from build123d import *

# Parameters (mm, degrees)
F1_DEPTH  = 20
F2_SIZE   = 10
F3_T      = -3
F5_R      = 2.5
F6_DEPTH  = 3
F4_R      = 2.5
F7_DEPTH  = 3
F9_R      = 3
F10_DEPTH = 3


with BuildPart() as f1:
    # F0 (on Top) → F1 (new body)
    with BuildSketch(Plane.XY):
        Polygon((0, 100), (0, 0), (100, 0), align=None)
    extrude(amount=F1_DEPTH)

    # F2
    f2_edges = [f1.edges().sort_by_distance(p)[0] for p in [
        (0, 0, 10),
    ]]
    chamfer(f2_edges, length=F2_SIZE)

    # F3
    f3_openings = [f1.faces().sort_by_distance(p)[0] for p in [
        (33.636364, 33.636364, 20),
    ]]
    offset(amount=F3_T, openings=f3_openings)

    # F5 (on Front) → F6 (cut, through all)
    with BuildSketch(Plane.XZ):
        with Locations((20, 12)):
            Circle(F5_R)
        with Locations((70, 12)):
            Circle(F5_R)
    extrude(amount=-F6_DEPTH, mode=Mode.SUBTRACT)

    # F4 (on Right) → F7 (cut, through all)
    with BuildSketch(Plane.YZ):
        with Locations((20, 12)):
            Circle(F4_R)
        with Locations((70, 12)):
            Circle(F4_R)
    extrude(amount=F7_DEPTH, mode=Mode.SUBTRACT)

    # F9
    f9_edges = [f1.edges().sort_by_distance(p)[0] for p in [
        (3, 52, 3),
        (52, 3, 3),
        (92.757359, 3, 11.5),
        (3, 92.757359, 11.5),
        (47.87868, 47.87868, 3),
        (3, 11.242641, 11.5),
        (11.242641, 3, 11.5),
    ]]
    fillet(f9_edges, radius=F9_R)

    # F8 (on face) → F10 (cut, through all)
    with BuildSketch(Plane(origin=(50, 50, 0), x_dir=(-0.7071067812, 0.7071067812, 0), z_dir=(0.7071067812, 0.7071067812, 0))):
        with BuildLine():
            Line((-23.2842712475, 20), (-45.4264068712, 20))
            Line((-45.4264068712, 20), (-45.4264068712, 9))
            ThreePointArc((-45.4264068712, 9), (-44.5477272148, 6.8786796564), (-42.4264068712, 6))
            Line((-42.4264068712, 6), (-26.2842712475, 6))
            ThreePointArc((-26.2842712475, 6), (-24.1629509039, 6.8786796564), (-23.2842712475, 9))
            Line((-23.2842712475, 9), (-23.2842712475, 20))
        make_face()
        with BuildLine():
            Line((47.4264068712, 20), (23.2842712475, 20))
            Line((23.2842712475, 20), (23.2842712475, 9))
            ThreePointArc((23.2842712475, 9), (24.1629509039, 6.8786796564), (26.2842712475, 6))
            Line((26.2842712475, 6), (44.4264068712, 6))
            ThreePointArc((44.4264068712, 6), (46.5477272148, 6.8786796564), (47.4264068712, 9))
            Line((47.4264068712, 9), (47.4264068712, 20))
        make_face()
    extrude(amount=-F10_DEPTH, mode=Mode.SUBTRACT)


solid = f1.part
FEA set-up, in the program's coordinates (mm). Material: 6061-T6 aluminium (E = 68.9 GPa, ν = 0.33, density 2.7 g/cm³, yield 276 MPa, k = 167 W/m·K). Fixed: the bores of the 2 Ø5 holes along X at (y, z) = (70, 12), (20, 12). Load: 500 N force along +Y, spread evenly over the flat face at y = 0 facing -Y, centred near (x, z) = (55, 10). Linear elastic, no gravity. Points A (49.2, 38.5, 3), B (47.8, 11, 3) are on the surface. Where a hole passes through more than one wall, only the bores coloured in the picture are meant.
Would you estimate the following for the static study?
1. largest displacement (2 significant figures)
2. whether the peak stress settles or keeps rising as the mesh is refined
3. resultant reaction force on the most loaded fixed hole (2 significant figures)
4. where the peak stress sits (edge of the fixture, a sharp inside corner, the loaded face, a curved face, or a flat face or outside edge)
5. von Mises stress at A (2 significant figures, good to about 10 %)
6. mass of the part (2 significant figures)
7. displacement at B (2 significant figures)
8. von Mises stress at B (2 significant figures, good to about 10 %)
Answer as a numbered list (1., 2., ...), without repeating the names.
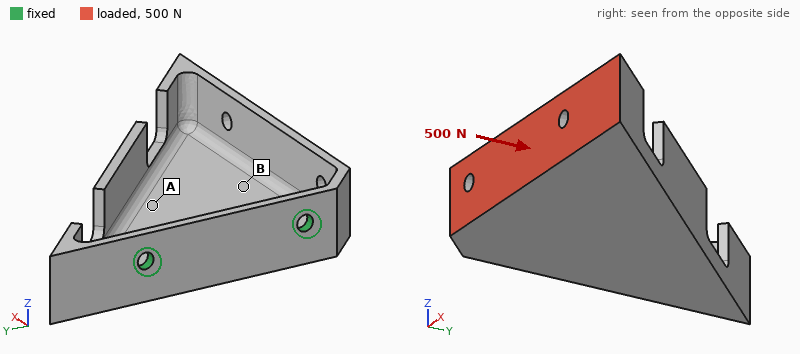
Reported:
1. 0.33 mm
2. keeps rising
3. 580 N
4. edge of the fixture
5. 6.4 MPa
6. 81 g
7. 0.097 mm
8. 22 MPa
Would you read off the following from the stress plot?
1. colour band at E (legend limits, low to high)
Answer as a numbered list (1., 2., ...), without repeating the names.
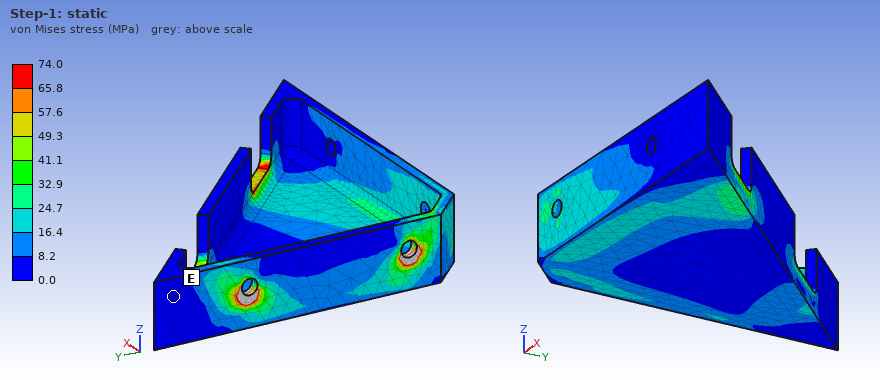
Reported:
1. 0.0 to 8.2 MPa
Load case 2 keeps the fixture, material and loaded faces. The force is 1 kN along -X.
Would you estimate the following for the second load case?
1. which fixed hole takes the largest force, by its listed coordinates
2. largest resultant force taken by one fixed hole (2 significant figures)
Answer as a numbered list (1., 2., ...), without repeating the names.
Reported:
1. (20, 12)
2. 1.3 kN
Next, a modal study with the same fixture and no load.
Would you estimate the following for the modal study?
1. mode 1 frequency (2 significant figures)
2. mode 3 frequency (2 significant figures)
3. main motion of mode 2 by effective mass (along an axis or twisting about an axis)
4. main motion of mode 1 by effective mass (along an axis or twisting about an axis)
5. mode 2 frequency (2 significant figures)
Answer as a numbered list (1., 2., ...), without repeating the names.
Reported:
1. 420 Hz
2. 2300 Hz
3. along Y
4. along Z
5. 1300 Hz
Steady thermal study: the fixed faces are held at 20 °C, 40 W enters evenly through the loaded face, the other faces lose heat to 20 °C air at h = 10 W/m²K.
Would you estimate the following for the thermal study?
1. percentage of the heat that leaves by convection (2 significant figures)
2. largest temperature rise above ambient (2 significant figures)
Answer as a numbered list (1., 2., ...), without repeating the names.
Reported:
1. 14 %
2. 74 K
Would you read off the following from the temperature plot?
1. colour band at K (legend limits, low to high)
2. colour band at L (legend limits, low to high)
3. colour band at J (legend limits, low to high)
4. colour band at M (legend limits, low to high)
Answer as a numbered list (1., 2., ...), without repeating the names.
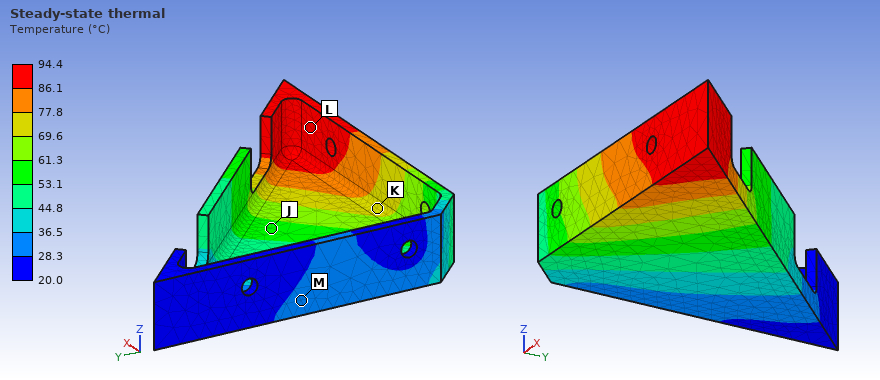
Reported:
1. 69.6 to 77.8 °C
2. 86.1 to 94.4 °C
3. 53.1 to 61.3 °C
4. 28.3 to 36.5 °C
